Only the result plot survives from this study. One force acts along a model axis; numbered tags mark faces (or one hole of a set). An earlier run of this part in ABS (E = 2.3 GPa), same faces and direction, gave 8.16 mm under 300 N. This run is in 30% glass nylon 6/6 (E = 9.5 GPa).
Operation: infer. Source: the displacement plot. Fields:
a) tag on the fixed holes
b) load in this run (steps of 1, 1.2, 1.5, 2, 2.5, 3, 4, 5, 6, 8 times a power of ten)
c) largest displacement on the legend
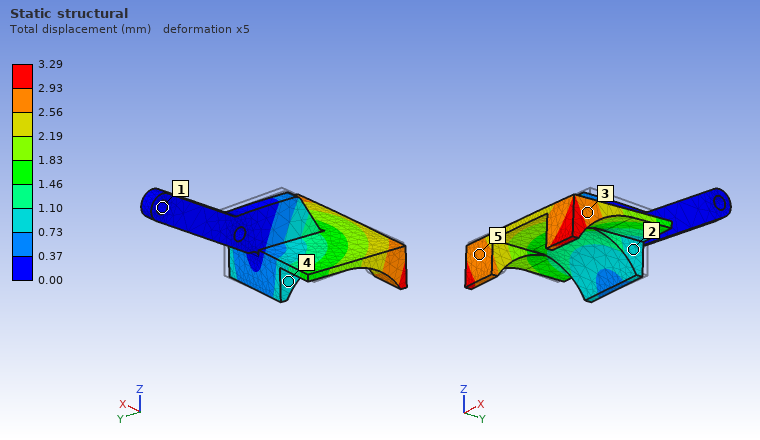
1
500 N
3.29 mm
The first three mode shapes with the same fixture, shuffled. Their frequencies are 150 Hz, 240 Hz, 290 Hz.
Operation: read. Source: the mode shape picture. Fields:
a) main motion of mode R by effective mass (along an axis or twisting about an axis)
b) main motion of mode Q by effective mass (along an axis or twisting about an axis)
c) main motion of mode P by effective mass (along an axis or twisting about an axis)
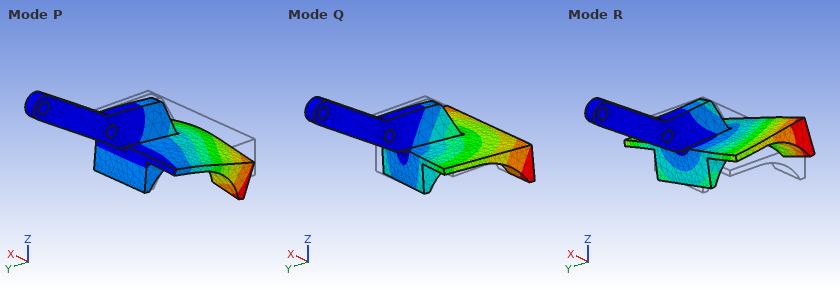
twisting about Y
along X
along Z
